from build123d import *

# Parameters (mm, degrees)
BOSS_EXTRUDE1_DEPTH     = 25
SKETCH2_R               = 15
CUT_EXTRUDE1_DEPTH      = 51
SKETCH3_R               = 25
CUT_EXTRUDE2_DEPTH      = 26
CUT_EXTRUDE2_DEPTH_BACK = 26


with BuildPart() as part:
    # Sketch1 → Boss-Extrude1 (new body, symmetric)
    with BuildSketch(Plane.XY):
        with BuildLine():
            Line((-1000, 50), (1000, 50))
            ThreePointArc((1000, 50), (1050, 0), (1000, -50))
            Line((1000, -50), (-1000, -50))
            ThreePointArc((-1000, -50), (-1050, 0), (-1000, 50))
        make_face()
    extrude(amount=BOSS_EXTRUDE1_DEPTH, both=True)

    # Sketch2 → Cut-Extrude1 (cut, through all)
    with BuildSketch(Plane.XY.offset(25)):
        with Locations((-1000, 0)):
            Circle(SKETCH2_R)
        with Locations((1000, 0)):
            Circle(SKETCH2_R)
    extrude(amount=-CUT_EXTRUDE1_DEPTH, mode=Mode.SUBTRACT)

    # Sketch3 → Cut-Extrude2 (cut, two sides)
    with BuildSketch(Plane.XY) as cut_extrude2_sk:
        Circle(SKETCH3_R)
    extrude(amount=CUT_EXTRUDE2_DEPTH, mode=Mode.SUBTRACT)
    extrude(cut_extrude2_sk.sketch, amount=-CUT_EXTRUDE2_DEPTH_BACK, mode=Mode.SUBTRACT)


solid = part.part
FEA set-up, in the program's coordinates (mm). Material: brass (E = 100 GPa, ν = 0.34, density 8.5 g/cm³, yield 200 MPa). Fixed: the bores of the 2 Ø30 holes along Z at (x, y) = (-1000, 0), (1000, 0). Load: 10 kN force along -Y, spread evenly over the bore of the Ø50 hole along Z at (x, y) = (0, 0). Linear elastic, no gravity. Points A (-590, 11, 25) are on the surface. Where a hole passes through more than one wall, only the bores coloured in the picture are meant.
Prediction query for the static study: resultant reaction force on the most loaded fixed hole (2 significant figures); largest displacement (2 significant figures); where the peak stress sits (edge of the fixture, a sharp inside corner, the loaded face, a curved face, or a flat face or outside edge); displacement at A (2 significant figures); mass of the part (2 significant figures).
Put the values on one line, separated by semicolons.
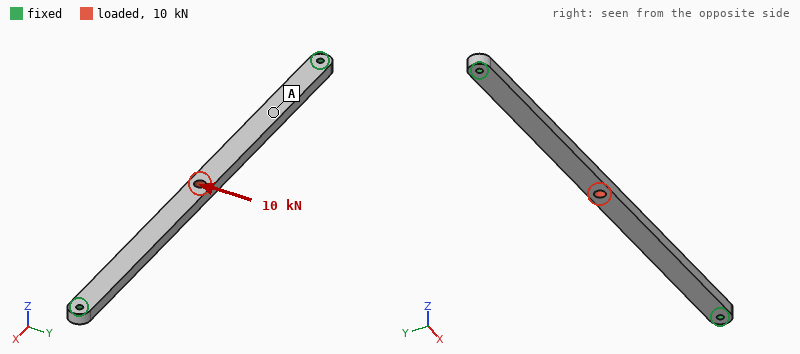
5.0 kN; 1.2 mm; edge of the fixture; 0.50 mm; 87 kg
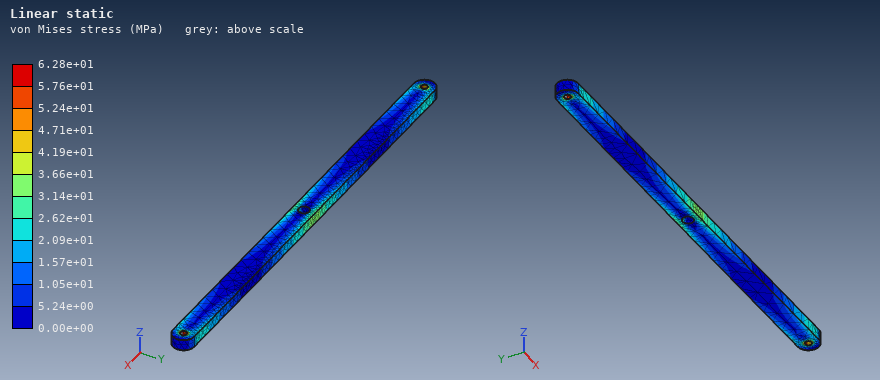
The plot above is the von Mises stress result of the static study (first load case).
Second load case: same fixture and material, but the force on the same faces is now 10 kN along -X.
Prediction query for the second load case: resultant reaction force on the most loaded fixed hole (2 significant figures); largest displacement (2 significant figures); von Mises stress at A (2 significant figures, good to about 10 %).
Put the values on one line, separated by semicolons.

5.0 kN; 10 µm; 1.0 MPa
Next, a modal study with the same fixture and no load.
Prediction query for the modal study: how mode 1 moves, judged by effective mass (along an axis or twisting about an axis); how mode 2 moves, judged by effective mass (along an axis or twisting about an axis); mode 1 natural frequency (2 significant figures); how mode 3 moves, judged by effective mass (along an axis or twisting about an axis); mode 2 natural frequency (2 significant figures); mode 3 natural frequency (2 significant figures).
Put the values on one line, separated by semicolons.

along Z; along Y; 44 Hz; twisting about Y; 79 Hz; 120 Hz
